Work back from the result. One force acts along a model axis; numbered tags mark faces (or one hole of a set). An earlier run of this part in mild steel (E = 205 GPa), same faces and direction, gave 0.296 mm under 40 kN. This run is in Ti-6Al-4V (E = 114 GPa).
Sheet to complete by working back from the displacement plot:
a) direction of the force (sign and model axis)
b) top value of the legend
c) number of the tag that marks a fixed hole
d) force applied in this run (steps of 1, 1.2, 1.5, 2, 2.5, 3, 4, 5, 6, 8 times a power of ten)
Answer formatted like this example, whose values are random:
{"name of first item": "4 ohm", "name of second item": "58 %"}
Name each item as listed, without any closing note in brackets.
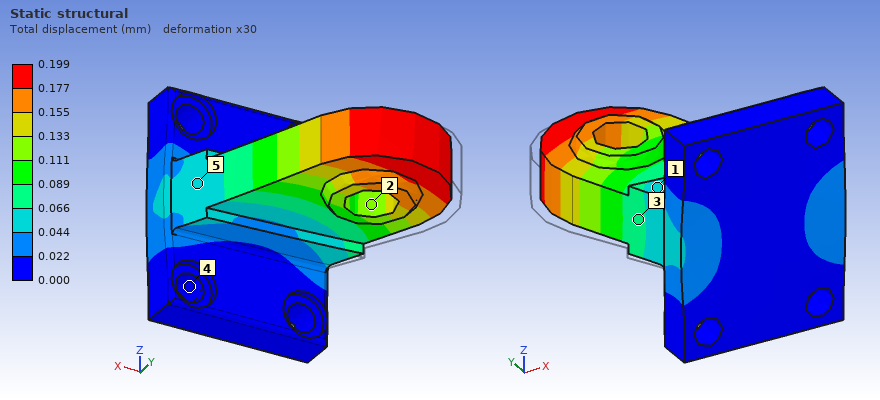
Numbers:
{"direction of the force": "+X", "top value of the legend": "0.199 mm", "number of the tag that marks a fixed hole": "4", "force applied in this run": "15 kN"}
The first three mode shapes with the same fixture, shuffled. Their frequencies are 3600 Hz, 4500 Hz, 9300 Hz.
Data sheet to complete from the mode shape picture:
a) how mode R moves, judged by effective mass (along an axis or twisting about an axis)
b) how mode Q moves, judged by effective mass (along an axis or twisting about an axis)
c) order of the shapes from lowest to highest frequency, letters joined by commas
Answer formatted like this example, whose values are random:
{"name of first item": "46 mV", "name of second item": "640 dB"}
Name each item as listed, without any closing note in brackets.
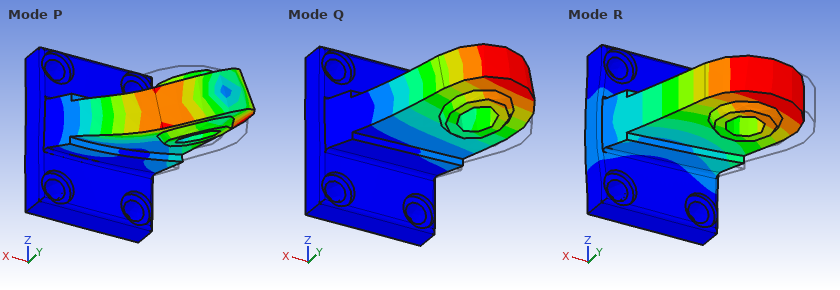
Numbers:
{"how mode R moves, judged by effective mass": "along X", "how mode Q moves, judged by effective mass": "along Z", "order of the shapes from lowest to highest frequency, letters joined by commas": "Q, R, P"}
